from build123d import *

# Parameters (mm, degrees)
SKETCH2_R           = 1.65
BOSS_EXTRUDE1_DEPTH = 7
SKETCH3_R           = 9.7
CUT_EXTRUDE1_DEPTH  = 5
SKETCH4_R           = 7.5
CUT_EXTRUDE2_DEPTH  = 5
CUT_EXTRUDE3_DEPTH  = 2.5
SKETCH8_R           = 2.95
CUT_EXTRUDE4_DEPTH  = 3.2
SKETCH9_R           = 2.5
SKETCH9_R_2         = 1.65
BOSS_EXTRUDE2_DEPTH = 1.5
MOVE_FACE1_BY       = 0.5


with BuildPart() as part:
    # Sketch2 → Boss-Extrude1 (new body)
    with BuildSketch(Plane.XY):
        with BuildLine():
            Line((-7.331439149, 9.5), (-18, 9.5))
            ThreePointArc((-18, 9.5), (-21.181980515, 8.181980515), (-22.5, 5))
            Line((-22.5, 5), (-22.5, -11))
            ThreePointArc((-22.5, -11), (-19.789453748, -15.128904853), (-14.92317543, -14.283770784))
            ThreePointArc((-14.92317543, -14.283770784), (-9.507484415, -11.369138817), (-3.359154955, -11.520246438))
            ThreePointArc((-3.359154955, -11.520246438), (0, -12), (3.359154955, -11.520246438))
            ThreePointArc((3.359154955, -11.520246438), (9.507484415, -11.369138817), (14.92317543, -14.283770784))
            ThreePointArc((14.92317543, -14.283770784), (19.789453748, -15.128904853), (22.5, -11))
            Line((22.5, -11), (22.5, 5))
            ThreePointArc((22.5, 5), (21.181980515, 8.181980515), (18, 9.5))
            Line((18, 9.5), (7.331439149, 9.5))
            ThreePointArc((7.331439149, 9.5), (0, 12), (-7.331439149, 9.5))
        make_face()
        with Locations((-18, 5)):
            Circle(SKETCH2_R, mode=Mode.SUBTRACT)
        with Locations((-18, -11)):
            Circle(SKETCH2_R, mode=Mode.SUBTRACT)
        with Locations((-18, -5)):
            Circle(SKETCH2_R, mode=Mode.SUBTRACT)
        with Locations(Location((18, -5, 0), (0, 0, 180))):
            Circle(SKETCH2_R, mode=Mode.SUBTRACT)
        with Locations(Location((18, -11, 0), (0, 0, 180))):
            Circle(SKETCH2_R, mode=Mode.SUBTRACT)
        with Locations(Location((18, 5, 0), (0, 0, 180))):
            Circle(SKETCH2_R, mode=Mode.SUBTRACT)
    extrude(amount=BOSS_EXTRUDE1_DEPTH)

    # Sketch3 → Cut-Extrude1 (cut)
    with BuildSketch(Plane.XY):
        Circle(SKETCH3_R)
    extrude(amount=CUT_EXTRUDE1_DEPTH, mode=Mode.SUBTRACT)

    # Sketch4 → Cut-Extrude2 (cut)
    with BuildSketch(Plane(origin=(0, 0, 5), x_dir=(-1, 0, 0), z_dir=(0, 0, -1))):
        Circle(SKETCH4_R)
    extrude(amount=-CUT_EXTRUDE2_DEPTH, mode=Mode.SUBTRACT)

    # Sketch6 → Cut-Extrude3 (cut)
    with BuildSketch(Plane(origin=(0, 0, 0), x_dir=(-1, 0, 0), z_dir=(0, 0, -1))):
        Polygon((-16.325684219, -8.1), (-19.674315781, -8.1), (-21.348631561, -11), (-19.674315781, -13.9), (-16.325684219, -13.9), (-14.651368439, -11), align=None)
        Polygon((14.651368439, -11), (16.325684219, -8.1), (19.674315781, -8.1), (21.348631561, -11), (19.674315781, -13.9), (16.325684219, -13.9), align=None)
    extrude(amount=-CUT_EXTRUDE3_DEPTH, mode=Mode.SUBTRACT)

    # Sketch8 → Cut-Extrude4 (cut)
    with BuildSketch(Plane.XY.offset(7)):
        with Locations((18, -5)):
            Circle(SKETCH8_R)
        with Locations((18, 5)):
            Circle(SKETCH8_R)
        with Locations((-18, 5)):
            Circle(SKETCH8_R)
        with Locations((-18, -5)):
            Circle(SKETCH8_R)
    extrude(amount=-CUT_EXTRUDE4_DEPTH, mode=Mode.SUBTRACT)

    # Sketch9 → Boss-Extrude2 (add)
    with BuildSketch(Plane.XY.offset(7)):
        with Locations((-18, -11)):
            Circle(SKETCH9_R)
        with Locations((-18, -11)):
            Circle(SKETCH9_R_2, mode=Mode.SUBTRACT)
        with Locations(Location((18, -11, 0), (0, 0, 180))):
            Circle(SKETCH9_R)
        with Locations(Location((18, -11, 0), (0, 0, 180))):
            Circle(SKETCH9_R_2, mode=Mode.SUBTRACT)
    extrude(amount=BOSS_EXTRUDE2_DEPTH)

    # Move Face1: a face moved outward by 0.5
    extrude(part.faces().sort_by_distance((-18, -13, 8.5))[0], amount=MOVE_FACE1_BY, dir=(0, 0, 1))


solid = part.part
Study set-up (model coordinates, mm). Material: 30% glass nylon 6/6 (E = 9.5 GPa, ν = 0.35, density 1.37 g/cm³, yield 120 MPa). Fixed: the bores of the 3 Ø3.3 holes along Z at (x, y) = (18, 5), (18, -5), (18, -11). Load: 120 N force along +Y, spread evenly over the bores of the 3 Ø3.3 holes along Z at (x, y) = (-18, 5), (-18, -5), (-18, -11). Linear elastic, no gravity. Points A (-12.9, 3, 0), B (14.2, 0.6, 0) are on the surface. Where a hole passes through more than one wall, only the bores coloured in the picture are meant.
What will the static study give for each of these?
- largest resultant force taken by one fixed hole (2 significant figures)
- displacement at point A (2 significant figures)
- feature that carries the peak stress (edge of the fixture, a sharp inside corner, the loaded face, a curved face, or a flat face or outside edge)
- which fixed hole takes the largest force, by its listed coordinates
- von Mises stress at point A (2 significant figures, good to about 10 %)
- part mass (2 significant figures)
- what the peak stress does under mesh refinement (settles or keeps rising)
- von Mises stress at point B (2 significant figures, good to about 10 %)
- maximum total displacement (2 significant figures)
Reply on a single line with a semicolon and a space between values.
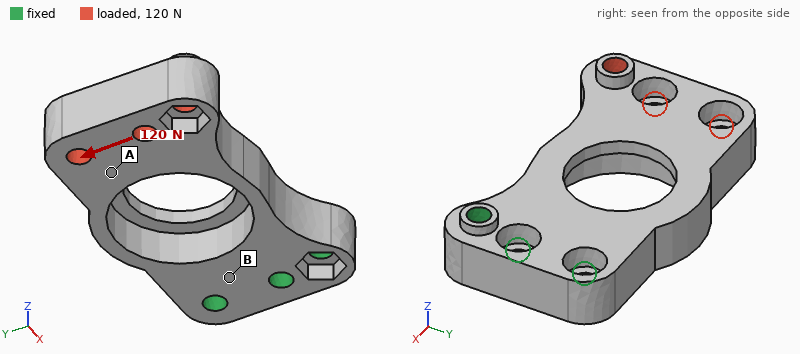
260 N; 0.18 mm; a sharp inside corner; (18, 5); 3.9 MPa; 6.4 g; keeps rising; 7.8 MPa; 0.21 mm
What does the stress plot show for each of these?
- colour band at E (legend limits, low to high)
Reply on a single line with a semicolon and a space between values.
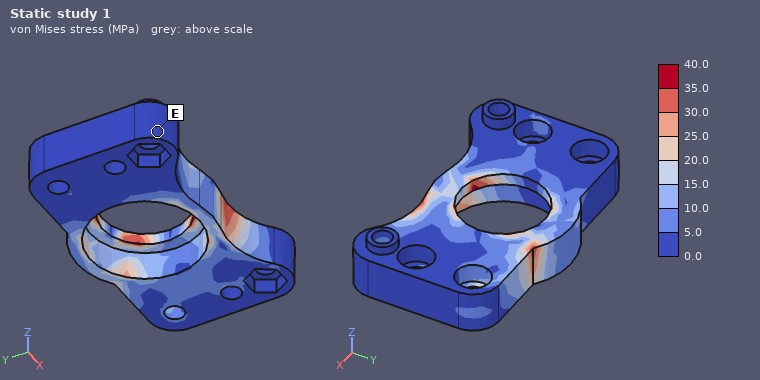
0.0 to 5.0 MPa
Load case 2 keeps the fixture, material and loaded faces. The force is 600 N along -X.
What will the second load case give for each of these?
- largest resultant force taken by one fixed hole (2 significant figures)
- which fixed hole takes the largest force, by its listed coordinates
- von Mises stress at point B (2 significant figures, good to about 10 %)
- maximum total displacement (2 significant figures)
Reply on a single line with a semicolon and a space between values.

310 N; (18, -11); 2.8 MPa; 0.12 mm
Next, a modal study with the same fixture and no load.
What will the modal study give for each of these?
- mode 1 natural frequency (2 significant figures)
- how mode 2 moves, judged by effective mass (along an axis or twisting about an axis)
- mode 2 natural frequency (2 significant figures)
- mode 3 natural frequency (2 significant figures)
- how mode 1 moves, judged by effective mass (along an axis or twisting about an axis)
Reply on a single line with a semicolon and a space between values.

1200 Hz; along Y; 2400 Hz; 4100 Hz; along Z
